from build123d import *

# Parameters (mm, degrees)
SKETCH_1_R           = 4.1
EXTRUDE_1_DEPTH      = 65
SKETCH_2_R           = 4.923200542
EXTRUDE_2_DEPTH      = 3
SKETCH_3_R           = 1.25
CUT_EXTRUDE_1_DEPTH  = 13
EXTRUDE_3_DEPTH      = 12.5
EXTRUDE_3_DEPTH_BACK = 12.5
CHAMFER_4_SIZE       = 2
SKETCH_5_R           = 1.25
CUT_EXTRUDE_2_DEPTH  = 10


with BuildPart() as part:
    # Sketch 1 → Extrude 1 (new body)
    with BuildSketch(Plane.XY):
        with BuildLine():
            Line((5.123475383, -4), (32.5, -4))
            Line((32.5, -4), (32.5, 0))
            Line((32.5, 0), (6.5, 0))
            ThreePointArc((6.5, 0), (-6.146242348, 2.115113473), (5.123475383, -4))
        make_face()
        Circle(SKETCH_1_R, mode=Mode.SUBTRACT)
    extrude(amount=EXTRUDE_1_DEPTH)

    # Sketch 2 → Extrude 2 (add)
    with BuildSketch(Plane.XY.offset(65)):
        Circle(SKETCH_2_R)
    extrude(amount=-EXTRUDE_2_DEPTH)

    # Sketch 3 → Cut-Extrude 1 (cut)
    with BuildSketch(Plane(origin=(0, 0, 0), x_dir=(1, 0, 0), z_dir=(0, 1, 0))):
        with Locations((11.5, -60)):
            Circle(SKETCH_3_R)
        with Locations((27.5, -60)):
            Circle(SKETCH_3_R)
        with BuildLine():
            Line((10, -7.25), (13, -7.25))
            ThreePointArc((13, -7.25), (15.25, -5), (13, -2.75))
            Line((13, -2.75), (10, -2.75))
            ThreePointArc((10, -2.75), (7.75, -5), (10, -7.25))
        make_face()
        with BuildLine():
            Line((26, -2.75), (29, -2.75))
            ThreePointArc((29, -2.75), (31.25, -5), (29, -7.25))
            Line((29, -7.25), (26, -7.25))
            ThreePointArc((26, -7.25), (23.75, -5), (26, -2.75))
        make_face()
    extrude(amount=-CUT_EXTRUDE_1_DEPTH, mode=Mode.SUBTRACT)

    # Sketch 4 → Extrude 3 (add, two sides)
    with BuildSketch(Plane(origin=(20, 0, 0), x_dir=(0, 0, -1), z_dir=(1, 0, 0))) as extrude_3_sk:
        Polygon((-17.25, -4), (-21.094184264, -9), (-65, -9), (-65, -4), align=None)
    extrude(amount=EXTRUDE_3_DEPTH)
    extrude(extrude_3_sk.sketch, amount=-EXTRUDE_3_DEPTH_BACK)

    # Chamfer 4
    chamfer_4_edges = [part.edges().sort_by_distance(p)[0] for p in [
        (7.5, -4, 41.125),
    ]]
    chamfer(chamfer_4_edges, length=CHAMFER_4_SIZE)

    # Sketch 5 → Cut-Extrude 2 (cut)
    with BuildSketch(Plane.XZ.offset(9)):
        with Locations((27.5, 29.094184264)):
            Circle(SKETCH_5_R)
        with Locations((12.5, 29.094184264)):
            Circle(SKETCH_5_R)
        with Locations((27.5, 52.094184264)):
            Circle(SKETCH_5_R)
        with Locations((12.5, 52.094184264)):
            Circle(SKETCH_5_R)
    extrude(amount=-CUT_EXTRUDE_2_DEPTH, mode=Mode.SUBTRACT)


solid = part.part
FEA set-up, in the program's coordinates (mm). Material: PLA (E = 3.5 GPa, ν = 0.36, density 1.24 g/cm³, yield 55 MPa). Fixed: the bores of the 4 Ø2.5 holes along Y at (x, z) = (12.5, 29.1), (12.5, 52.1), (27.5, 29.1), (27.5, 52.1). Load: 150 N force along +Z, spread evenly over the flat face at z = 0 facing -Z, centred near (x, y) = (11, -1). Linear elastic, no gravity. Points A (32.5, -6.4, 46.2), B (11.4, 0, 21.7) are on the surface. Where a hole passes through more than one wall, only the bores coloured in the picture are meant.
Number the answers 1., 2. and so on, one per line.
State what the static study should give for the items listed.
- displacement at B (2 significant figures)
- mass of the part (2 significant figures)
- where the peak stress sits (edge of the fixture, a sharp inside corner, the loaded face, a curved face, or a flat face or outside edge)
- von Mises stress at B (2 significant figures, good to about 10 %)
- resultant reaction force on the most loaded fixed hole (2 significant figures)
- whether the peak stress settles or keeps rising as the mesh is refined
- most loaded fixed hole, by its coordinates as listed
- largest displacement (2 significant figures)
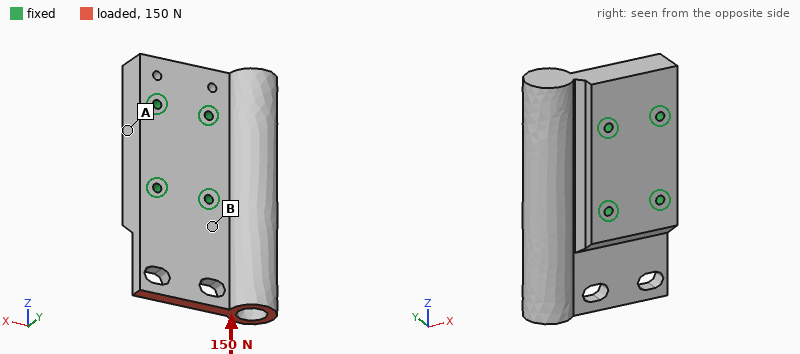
1. 4.3 µm
2. 22 g
3. a sharp inside corner
4. 1.2 MPa
5. 87 N
6. keeps rising
7. (12.5, 29.1)
8. 19 µm
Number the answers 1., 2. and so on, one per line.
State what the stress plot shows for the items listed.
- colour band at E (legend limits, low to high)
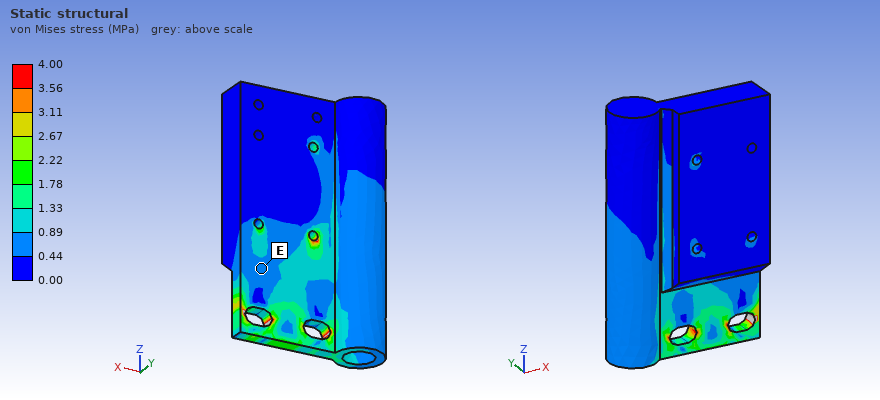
1. 0.44 to 0.89 MPa
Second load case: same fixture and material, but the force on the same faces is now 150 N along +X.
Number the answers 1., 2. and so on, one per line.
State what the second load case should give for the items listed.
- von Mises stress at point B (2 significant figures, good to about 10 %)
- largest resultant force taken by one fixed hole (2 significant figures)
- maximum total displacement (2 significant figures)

1. 2.1 MPa
2. 190 N
3. 93 µm
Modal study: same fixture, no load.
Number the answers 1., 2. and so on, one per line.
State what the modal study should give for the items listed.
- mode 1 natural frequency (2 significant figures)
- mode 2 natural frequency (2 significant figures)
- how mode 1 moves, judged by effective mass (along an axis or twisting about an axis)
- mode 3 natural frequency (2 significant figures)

1. 2400 Hz
2. 3100 Hz
3. along Y
4. 4000 Hz
